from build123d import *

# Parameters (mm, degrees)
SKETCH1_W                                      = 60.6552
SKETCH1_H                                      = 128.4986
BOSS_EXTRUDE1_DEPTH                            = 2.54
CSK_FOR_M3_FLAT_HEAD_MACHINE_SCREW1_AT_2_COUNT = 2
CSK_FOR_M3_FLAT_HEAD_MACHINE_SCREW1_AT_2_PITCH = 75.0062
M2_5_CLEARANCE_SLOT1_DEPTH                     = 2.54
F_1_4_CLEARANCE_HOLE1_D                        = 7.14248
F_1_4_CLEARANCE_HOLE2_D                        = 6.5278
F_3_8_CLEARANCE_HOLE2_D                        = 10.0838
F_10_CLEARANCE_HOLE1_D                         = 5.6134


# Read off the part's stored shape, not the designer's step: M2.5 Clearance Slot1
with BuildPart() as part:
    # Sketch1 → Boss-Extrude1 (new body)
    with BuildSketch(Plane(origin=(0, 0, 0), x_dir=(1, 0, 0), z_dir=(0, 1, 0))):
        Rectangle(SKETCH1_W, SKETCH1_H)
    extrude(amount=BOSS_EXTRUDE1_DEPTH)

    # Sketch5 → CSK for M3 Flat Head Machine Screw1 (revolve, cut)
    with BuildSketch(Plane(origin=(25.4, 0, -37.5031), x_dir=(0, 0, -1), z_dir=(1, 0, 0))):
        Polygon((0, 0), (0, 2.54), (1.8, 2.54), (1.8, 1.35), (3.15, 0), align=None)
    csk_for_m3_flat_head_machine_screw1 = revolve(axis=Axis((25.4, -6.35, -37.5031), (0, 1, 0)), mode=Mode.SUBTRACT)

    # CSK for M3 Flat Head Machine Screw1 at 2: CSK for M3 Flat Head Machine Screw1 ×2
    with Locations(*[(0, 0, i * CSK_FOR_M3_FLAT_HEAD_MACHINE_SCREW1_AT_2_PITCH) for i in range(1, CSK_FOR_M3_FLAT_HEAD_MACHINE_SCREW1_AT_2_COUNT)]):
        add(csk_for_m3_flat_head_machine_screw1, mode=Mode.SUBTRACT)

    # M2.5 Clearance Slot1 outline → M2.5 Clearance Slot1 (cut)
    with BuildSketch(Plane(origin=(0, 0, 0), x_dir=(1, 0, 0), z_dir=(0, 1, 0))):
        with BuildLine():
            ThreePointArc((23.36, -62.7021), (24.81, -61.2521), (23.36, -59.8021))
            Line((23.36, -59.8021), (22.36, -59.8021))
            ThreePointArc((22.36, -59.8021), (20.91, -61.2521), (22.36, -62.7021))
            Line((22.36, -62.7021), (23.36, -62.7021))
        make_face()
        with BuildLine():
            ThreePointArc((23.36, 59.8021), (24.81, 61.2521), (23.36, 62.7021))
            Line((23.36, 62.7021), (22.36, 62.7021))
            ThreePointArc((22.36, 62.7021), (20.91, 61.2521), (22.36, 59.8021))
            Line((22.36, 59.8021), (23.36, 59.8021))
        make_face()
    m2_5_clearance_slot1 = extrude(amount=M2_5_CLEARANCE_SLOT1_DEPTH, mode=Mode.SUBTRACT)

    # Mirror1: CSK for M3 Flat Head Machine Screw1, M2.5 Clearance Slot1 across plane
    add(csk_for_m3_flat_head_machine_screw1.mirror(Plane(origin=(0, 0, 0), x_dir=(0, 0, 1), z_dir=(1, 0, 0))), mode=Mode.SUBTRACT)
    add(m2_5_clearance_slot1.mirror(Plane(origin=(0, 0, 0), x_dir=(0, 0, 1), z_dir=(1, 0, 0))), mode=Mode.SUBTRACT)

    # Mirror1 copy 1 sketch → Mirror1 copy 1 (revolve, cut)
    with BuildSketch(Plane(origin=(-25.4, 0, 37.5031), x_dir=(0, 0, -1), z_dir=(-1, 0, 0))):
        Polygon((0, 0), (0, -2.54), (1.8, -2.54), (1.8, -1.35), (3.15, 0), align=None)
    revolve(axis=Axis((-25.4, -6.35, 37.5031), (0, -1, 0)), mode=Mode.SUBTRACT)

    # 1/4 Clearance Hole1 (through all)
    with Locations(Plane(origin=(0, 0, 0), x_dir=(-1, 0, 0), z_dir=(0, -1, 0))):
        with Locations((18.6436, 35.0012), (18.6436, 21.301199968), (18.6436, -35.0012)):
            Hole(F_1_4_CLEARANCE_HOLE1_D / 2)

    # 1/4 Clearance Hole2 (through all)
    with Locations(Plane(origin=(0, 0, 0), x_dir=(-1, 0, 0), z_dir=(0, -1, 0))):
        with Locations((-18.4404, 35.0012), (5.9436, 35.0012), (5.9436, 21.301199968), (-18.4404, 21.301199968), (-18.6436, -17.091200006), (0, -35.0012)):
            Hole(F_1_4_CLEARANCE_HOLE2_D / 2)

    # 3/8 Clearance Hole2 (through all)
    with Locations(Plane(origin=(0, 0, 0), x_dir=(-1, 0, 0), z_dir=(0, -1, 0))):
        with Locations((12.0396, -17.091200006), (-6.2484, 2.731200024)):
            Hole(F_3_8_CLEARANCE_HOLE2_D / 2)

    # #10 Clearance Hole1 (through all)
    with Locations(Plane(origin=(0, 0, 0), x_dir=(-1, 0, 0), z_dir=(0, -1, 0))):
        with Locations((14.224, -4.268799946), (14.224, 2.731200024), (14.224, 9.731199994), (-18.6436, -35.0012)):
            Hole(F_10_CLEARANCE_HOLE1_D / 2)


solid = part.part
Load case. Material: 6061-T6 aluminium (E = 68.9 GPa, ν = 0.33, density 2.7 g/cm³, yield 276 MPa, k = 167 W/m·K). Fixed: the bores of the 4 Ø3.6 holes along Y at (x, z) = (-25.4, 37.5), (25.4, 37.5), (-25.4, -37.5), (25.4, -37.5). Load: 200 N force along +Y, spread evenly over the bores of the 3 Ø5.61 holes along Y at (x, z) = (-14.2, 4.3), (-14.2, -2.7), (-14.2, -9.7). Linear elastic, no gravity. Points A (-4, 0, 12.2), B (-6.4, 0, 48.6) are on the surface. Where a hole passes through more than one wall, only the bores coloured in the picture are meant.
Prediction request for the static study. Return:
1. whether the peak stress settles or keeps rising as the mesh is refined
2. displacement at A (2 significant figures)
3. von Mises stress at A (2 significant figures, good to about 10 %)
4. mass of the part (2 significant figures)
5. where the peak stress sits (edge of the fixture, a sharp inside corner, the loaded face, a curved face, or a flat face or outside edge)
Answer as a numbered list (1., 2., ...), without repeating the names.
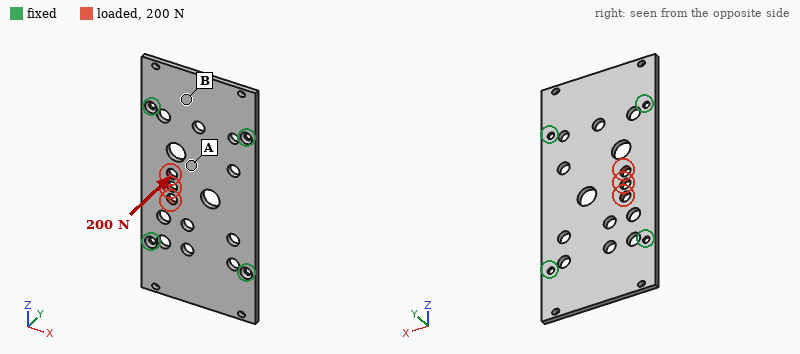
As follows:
1. keeps rising
2. 0.13 mm
3. 20 MPa
4. 49 g
5. edge of the fixture
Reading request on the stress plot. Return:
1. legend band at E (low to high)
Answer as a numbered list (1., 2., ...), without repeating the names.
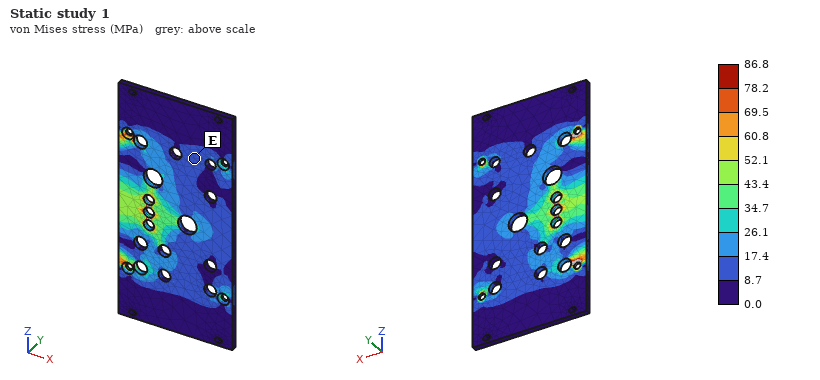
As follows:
1. 8.7 to 17.4 MPa
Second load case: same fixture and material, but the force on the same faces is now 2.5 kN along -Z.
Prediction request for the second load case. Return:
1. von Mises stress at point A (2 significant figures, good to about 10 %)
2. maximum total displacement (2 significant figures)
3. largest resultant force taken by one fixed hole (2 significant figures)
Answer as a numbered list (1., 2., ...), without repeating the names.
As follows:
1. 15 MPa
2. 20 µm
3. 860 N
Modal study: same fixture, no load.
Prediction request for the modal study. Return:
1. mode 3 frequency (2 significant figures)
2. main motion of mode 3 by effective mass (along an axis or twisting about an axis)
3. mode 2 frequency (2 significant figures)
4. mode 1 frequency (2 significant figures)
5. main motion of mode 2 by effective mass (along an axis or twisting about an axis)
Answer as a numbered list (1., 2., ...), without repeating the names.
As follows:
1. 2000 Hz
2. along Y
3. 1900 Hz
4. 1600 Hz
5. twisting about X
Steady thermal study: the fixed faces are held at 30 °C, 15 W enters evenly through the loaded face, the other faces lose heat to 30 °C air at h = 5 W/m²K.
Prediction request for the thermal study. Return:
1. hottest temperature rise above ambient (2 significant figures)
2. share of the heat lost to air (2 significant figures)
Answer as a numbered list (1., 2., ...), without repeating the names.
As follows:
1. 24 K
2. 3.6 %
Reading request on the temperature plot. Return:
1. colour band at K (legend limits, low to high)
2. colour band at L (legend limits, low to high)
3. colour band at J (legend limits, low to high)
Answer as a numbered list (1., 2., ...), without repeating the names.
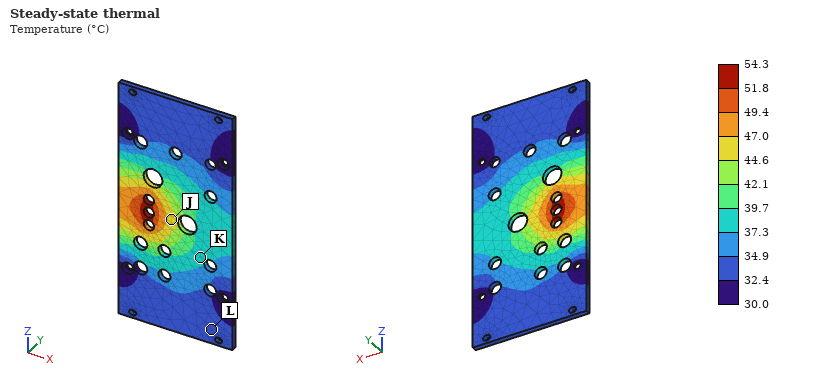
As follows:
1. 37.3 to 39.7 °C
2. 32.4 to 34.9 °C
3. 44.6 to 47.0 °C
